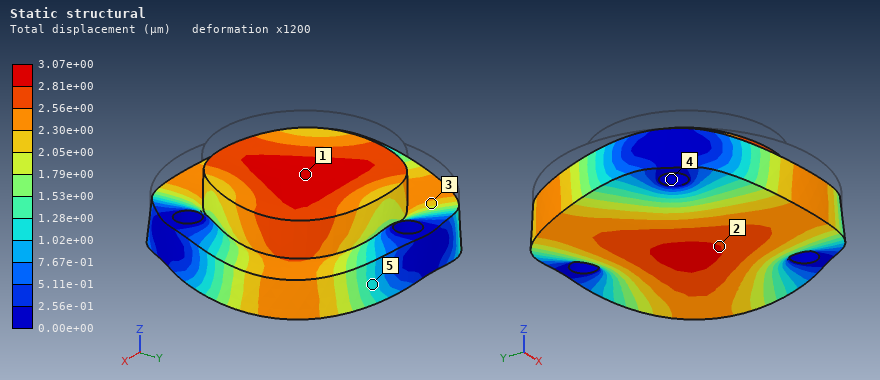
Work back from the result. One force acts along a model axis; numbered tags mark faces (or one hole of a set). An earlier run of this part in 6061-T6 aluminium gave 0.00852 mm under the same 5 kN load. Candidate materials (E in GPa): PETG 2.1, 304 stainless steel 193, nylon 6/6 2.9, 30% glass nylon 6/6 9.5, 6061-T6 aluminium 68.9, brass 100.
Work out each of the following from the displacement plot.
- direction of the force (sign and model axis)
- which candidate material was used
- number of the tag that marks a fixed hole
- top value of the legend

-Z
304 stainless steel
4
3.07e+00 µm
